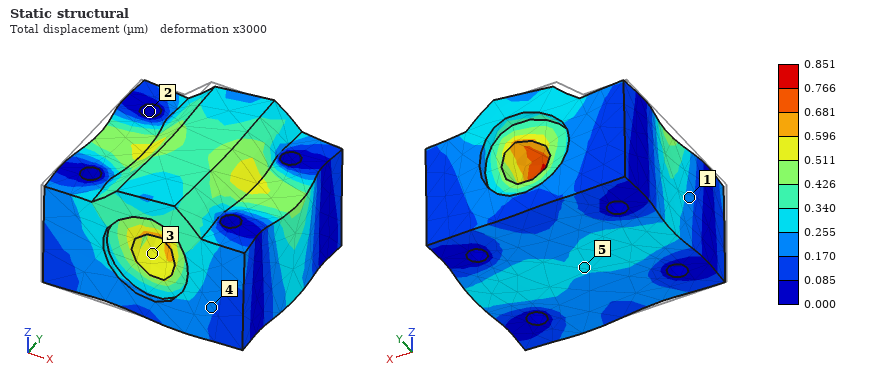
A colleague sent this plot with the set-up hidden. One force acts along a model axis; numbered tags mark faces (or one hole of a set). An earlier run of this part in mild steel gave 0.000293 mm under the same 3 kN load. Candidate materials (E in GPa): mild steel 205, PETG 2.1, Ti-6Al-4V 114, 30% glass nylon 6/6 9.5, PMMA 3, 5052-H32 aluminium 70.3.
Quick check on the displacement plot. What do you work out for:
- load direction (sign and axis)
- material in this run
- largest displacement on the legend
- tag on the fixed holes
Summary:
+X
5052-H32 aluminium
0.851 µm
2
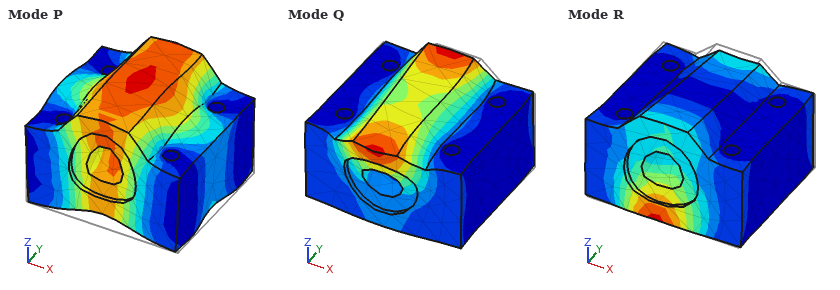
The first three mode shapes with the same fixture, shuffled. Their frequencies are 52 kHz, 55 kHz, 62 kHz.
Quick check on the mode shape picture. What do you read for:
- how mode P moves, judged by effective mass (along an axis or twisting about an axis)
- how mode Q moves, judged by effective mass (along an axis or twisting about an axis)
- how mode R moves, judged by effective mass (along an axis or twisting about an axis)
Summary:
along Z
along Y
along Y
